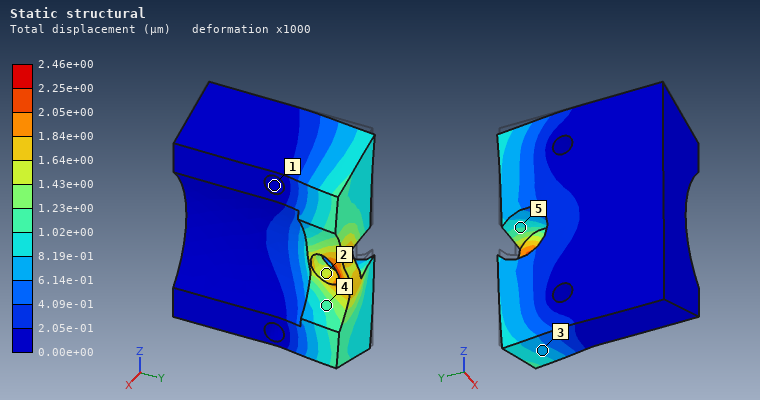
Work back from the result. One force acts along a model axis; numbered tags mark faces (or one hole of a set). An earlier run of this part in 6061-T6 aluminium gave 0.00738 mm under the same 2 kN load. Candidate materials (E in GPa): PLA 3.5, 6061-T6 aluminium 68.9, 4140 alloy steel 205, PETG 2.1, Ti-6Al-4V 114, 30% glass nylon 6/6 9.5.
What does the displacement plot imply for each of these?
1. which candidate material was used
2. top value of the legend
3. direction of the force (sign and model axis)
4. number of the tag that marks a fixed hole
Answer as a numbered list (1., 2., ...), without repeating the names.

1. 4140 alloy steel
2. 2.46e+00 µm
3. -Z
4. 1
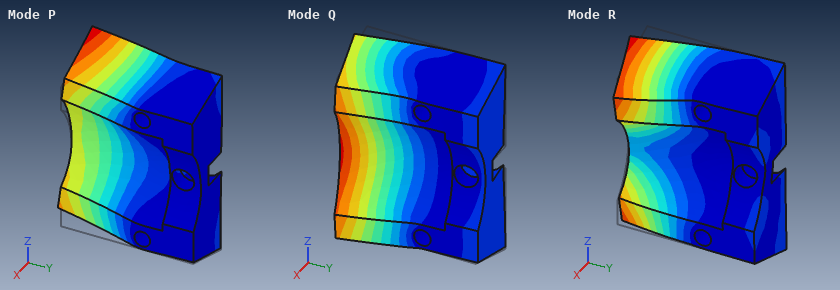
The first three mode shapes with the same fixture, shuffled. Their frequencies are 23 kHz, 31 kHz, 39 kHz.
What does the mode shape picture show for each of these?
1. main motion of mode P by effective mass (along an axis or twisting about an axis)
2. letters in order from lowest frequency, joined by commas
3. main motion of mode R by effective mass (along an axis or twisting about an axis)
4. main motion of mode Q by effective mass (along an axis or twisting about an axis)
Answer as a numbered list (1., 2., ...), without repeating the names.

1. along Z
2. Q, R, P
3. twisting about Y
4. along X
